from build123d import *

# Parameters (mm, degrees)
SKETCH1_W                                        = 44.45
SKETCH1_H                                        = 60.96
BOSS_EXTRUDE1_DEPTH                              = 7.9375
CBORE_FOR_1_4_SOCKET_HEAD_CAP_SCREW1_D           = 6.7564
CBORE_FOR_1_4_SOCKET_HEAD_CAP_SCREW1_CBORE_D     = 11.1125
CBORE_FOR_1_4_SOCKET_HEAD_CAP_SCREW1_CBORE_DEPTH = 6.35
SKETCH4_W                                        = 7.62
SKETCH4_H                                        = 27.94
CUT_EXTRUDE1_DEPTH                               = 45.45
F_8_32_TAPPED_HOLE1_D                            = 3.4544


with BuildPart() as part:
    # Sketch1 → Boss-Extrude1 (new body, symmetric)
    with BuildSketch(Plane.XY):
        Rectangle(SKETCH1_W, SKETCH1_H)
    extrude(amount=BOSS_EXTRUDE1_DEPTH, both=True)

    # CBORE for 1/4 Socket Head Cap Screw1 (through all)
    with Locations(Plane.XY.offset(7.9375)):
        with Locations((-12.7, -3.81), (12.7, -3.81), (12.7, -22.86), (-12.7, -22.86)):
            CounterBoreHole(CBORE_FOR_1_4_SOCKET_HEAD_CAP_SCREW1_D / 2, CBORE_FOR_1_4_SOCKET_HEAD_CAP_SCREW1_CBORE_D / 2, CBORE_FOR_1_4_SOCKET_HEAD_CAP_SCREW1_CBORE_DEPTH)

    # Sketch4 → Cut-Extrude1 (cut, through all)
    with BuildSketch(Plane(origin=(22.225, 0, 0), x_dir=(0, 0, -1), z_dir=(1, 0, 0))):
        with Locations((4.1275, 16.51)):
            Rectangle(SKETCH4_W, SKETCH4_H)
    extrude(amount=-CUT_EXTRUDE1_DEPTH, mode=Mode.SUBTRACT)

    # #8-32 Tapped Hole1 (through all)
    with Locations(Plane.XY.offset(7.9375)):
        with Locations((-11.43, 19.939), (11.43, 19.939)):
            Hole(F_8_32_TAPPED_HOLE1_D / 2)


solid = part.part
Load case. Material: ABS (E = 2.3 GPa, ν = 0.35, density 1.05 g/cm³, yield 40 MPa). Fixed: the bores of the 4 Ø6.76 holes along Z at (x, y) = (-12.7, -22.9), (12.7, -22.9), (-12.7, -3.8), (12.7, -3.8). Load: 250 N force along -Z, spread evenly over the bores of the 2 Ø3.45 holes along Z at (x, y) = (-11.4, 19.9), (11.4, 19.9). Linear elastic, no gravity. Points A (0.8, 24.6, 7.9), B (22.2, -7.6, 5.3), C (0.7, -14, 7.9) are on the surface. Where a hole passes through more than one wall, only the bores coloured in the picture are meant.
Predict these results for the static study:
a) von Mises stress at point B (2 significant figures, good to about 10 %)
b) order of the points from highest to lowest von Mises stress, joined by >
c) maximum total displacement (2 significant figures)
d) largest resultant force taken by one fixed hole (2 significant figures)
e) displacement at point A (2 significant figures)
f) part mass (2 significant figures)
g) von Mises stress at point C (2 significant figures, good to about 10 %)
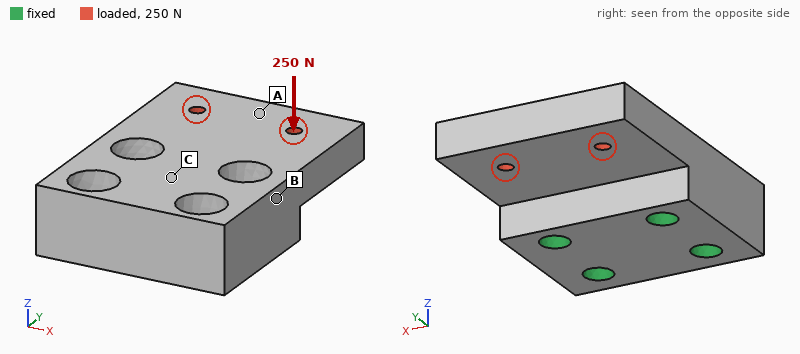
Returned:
3.3 MPa
B > C > A
0.42 mm
250 N
0.33 mm
31 g
1.8 MPa
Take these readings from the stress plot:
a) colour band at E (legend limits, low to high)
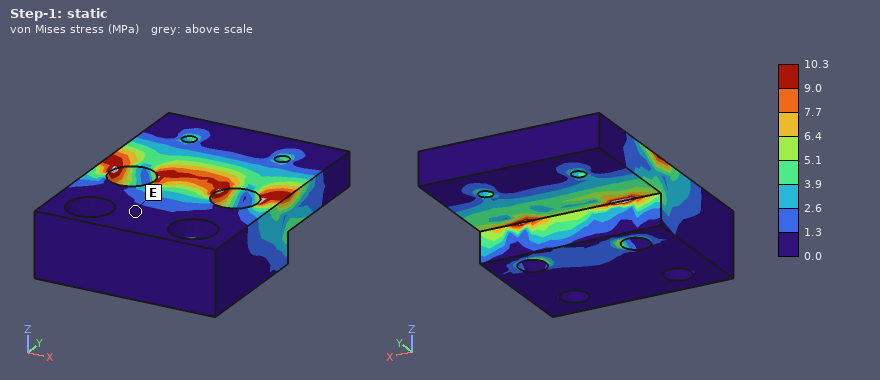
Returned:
0.0 to 1.3 MPa
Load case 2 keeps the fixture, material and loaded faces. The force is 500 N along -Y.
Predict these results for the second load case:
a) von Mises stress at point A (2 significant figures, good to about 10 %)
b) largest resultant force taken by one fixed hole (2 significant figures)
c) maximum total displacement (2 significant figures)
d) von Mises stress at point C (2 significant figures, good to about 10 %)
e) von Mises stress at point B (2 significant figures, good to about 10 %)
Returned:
0.49 MPa
180 N
73 µm
0.92 MPa
1.7 MPa
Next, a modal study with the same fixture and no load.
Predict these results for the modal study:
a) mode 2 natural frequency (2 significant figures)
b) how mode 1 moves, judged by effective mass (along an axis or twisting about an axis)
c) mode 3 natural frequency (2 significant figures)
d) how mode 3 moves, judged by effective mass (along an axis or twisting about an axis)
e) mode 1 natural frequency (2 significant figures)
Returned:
3000 Hz
along Z
4300 Hz
along X
1600 Hz
